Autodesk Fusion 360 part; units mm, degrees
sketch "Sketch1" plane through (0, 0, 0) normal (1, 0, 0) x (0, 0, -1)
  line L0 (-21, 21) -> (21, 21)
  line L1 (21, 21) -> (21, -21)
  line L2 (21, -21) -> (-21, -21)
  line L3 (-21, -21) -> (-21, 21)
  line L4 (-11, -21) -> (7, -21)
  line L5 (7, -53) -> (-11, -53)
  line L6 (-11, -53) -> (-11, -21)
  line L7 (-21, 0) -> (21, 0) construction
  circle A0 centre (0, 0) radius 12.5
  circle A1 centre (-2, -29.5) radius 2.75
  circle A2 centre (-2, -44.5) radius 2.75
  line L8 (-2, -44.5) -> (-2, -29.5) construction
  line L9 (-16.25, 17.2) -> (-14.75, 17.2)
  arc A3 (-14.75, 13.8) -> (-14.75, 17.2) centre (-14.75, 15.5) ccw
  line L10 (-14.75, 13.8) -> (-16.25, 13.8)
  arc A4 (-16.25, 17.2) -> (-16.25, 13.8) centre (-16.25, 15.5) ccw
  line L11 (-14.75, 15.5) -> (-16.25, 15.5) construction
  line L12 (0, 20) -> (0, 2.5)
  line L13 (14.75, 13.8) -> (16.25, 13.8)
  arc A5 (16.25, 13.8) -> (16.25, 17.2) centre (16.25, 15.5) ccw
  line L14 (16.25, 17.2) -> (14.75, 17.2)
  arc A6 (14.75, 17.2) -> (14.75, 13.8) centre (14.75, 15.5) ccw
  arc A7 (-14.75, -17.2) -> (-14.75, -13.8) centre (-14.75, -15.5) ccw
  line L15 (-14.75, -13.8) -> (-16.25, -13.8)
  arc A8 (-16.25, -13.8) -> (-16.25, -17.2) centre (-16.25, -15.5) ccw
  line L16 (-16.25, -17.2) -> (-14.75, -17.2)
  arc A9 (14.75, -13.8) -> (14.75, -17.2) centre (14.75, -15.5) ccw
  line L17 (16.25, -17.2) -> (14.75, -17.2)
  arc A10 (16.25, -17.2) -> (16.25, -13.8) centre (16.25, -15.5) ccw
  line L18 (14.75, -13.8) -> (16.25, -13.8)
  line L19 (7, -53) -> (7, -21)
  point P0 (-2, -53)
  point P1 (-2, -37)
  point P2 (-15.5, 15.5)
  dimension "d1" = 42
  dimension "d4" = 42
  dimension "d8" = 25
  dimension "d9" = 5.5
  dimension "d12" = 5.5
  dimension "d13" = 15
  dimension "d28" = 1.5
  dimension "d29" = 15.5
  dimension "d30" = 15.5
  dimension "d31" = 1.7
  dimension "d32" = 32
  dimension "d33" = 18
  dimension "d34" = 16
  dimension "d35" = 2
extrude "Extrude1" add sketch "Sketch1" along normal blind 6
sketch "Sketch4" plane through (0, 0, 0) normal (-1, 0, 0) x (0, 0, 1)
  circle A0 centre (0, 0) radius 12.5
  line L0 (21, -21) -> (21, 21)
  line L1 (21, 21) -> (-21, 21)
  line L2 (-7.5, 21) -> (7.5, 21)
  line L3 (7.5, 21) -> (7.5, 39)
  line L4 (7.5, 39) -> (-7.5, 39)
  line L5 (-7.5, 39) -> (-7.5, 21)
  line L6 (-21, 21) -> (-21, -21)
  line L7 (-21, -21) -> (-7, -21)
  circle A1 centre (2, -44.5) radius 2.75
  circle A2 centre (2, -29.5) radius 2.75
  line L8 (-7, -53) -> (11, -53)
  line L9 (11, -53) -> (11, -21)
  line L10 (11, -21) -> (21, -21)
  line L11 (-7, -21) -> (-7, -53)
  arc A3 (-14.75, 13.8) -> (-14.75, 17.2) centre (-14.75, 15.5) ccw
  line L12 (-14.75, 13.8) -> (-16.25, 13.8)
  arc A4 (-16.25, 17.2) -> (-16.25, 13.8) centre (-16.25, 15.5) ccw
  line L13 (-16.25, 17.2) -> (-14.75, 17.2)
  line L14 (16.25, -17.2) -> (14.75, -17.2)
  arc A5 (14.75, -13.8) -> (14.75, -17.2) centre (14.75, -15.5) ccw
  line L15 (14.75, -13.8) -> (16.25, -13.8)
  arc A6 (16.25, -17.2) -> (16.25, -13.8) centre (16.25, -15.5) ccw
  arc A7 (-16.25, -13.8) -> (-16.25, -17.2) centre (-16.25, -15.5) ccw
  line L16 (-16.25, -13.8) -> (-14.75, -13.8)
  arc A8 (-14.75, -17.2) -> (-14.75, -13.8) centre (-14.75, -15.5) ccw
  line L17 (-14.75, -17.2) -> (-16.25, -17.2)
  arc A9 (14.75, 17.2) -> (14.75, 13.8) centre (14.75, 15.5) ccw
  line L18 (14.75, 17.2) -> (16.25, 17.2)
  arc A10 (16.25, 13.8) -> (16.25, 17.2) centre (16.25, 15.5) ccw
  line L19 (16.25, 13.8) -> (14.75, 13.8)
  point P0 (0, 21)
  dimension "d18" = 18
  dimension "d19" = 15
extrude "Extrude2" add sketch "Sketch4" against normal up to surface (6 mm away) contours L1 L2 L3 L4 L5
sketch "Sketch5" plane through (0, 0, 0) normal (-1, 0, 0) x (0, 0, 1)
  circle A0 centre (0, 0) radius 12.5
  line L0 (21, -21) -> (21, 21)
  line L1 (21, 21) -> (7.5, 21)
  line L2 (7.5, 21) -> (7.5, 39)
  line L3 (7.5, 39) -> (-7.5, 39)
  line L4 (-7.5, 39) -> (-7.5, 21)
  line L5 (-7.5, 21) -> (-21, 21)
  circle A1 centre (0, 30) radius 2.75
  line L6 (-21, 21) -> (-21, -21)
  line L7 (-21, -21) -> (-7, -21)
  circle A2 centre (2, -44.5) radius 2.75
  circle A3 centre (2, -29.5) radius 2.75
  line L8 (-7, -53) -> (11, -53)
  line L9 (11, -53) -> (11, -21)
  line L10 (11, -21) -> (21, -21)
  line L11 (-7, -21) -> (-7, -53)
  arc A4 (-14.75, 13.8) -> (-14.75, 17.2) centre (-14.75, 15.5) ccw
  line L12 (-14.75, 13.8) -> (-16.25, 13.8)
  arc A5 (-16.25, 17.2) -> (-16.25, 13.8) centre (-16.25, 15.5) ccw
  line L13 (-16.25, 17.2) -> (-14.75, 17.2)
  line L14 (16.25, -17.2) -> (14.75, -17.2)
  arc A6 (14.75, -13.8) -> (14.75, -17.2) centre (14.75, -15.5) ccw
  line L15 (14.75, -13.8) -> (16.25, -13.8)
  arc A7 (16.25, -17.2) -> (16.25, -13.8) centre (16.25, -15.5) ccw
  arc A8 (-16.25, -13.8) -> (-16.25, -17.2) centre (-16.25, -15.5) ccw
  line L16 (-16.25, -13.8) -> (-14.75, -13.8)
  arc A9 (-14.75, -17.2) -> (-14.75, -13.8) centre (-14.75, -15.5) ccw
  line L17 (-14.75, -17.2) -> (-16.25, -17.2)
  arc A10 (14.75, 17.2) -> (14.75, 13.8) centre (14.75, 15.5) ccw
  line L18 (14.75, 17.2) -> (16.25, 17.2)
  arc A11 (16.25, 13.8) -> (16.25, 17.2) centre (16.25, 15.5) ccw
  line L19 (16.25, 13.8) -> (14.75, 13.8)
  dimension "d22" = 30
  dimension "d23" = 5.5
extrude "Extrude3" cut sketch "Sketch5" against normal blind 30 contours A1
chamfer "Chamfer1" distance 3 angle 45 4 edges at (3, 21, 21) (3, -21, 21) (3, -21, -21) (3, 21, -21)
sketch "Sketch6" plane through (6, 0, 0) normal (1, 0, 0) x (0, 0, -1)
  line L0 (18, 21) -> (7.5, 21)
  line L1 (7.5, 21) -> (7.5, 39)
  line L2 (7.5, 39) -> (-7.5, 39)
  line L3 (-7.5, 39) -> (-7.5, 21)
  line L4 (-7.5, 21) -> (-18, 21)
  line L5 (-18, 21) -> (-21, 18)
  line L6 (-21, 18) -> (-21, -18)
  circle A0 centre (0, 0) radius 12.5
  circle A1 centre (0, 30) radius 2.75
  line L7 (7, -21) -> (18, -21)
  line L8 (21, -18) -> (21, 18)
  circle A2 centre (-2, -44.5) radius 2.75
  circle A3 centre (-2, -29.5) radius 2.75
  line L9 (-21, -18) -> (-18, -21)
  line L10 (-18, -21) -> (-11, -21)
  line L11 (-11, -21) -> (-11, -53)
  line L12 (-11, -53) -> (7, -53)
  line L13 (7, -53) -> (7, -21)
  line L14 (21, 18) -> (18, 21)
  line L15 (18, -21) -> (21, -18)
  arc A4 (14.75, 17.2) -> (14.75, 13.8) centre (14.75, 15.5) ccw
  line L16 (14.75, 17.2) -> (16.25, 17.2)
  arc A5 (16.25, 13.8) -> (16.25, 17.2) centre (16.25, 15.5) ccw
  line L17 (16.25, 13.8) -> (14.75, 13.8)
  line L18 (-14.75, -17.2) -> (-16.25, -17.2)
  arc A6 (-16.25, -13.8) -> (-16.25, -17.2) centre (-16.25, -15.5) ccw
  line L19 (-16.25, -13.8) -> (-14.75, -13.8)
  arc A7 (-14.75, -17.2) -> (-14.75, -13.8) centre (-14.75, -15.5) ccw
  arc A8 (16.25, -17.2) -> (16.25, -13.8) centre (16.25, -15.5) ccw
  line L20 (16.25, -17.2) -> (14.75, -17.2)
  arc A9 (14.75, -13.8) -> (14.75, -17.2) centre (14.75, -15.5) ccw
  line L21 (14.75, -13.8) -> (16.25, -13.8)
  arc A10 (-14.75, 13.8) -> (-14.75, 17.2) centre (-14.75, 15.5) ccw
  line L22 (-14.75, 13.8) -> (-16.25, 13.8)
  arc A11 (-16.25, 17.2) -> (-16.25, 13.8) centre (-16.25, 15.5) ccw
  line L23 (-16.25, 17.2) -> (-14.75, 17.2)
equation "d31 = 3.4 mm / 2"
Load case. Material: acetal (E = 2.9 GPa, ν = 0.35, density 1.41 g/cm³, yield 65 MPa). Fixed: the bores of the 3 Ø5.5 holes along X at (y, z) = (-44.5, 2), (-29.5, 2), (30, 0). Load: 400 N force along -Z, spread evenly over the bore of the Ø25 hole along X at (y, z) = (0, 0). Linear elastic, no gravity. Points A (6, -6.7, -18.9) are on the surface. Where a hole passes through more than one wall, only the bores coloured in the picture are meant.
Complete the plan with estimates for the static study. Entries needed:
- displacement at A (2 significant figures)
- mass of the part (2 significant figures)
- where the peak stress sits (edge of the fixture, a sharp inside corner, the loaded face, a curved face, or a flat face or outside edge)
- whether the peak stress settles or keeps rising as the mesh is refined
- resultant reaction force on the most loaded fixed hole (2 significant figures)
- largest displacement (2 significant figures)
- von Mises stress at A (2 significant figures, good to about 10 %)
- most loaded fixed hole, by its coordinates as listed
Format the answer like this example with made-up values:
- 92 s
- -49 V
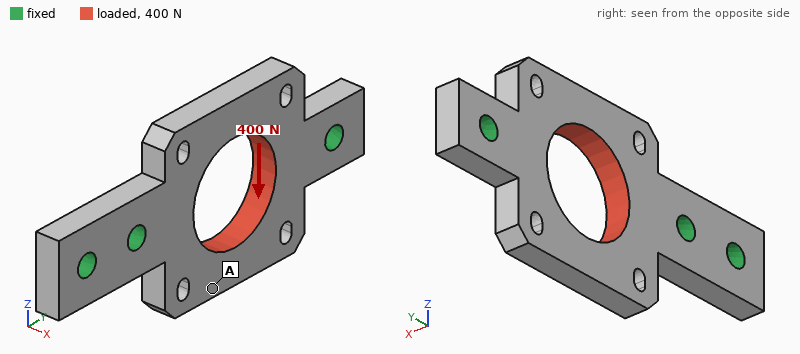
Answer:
- 42 µm
- 17 g
- edge of the fixture
- keeps rising
- 240 N
- 50 µm
- 1.4 MPa
- (-29.5, 2)
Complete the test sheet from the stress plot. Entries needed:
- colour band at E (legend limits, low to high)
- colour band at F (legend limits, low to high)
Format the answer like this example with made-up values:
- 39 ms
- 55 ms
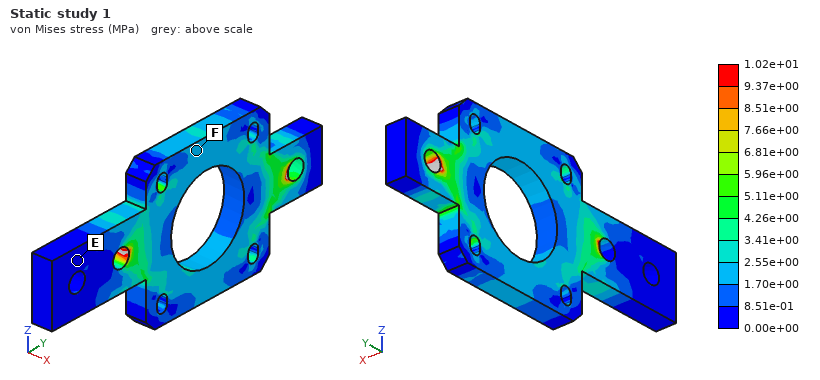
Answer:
- 0.00e+00 to 8.51e-01 MPa
- 1.70e+00 to 2.55e+00 MPa
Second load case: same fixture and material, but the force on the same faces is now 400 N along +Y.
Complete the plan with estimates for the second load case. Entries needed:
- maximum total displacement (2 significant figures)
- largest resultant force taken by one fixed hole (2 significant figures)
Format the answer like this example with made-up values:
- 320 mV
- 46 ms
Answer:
- 26 µm
- 190 N
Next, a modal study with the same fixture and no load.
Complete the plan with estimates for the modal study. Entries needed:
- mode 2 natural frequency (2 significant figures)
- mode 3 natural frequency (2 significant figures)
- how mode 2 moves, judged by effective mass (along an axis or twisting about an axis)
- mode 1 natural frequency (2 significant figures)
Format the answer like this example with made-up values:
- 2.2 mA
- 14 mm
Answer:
- 1800 Hz
- 3400 Hz
- along X
- 1400 Hz
